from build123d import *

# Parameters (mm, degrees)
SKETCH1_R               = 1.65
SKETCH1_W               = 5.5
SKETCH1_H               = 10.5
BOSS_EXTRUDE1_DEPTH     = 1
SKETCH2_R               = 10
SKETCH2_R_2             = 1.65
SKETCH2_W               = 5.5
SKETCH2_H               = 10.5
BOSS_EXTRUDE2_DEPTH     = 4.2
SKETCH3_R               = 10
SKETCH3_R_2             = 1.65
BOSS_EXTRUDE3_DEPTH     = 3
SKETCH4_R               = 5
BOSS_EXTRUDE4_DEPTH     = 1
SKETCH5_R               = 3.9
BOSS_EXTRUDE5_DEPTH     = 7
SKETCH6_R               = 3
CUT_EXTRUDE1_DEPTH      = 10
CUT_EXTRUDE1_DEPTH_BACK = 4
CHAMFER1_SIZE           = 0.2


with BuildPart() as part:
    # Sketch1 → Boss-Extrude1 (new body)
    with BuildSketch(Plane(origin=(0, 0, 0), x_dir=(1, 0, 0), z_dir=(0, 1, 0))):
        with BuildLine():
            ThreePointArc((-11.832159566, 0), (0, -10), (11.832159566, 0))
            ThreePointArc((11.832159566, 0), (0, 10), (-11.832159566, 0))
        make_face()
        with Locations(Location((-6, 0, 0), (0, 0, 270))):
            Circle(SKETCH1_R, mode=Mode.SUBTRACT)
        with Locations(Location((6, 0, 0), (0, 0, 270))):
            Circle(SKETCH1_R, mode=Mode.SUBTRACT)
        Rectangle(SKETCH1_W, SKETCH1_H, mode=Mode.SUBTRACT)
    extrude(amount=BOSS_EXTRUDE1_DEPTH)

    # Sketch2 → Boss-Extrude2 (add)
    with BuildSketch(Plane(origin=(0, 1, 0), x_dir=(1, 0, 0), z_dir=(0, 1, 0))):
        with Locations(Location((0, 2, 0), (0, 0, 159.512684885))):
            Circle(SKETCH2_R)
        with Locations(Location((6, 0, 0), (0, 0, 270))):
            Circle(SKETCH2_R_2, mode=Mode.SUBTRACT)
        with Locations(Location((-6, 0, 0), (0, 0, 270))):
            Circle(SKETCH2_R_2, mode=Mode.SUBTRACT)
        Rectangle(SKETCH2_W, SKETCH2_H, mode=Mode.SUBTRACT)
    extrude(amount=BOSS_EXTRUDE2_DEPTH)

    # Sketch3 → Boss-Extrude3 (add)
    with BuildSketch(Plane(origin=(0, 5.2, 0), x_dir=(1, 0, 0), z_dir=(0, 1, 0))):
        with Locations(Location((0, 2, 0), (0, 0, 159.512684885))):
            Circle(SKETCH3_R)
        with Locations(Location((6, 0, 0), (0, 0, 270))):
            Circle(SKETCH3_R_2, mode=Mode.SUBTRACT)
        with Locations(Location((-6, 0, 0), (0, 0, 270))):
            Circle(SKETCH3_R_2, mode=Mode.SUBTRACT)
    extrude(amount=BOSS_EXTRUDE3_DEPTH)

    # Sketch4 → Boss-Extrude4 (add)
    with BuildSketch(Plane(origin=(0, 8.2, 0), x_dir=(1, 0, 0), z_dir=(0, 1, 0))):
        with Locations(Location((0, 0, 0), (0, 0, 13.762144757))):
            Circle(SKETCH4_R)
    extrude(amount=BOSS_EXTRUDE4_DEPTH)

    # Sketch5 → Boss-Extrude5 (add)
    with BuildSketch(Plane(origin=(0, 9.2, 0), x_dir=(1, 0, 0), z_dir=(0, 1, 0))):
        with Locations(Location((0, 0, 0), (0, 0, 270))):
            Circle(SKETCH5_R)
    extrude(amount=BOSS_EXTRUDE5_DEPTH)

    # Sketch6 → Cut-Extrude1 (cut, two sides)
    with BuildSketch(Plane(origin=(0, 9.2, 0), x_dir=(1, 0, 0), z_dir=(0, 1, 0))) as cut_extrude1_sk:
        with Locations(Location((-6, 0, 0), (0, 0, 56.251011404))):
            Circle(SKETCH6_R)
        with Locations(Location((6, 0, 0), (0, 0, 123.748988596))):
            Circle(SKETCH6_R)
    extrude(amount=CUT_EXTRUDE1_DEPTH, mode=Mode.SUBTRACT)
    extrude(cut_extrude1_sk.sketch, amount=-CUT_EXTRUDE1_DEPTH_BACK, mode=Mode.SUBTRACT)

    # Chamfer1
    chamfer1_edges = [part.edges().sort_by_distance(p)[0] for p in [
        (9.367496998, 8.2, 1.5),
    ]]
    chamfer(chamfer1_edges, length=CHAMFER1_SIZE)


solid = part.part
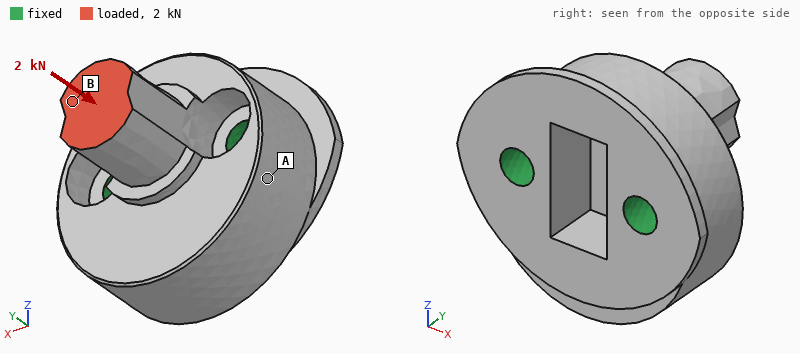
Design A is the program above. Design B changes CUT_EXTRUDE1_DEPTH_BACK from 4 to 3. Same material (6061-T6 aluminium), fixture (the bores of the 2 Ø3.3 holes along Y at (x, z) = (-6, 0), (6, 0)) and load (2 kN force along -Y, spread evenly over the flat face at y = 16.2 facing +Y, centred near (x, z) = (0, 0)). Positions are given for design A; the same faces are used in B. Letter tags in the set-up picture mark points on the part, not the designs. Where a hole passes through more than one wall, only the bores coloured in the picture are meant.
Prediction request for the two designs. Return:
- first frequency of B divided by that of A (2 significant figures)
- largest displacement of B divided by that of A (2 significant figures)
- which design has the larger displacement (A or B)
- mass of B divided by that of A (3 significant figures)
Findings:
1.2
0.91
A
1.02
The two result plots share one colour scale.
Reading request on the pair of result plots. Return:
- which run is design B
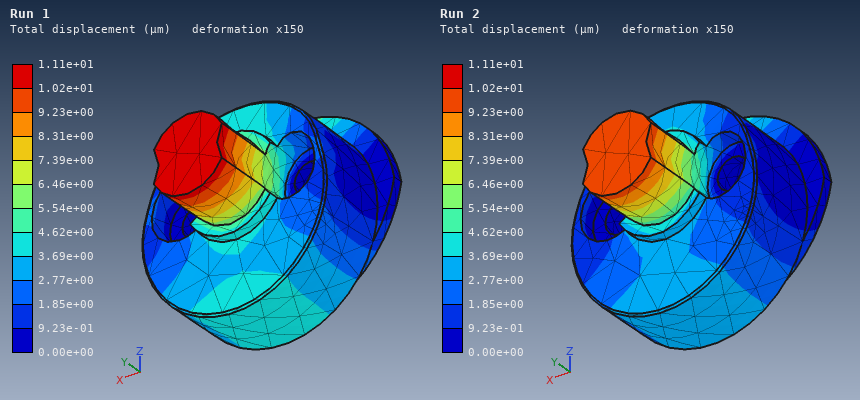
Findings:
Run 2
